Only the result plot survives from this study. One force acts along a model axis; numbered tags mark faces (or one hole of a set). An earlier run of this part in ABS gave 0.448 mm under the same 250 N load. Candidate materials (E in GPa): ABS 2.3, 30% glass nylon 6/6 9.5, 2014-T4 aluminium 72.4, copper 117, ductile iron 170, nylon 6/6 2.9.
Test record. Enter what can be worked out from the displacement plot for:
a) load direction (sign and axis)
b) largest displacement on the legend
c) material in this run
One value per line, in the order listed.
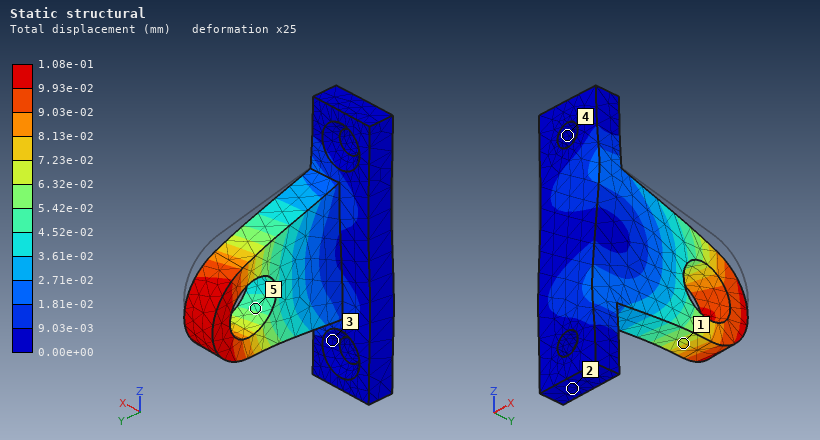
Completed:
-Z
1.08e-01 mm
30% glass nylon 6/6
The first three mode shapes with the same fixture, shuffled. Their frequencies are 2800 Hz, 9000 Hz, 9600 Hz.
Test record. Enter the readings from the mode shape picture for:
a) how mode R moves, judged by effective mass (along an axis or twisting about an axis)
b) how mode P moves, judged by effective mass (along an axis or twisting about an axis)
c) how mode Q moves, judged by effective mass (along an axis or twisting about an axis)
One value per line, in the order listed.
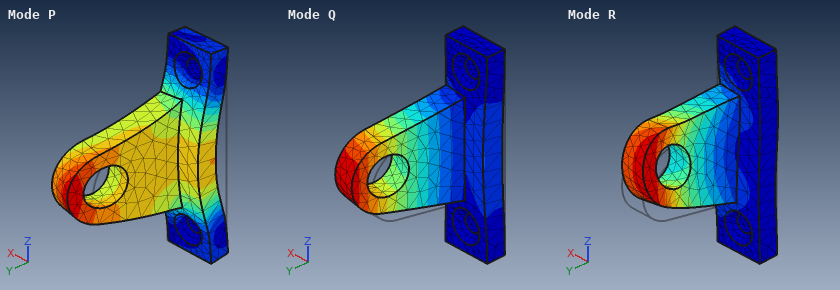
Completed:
along Z
along Y
along X
